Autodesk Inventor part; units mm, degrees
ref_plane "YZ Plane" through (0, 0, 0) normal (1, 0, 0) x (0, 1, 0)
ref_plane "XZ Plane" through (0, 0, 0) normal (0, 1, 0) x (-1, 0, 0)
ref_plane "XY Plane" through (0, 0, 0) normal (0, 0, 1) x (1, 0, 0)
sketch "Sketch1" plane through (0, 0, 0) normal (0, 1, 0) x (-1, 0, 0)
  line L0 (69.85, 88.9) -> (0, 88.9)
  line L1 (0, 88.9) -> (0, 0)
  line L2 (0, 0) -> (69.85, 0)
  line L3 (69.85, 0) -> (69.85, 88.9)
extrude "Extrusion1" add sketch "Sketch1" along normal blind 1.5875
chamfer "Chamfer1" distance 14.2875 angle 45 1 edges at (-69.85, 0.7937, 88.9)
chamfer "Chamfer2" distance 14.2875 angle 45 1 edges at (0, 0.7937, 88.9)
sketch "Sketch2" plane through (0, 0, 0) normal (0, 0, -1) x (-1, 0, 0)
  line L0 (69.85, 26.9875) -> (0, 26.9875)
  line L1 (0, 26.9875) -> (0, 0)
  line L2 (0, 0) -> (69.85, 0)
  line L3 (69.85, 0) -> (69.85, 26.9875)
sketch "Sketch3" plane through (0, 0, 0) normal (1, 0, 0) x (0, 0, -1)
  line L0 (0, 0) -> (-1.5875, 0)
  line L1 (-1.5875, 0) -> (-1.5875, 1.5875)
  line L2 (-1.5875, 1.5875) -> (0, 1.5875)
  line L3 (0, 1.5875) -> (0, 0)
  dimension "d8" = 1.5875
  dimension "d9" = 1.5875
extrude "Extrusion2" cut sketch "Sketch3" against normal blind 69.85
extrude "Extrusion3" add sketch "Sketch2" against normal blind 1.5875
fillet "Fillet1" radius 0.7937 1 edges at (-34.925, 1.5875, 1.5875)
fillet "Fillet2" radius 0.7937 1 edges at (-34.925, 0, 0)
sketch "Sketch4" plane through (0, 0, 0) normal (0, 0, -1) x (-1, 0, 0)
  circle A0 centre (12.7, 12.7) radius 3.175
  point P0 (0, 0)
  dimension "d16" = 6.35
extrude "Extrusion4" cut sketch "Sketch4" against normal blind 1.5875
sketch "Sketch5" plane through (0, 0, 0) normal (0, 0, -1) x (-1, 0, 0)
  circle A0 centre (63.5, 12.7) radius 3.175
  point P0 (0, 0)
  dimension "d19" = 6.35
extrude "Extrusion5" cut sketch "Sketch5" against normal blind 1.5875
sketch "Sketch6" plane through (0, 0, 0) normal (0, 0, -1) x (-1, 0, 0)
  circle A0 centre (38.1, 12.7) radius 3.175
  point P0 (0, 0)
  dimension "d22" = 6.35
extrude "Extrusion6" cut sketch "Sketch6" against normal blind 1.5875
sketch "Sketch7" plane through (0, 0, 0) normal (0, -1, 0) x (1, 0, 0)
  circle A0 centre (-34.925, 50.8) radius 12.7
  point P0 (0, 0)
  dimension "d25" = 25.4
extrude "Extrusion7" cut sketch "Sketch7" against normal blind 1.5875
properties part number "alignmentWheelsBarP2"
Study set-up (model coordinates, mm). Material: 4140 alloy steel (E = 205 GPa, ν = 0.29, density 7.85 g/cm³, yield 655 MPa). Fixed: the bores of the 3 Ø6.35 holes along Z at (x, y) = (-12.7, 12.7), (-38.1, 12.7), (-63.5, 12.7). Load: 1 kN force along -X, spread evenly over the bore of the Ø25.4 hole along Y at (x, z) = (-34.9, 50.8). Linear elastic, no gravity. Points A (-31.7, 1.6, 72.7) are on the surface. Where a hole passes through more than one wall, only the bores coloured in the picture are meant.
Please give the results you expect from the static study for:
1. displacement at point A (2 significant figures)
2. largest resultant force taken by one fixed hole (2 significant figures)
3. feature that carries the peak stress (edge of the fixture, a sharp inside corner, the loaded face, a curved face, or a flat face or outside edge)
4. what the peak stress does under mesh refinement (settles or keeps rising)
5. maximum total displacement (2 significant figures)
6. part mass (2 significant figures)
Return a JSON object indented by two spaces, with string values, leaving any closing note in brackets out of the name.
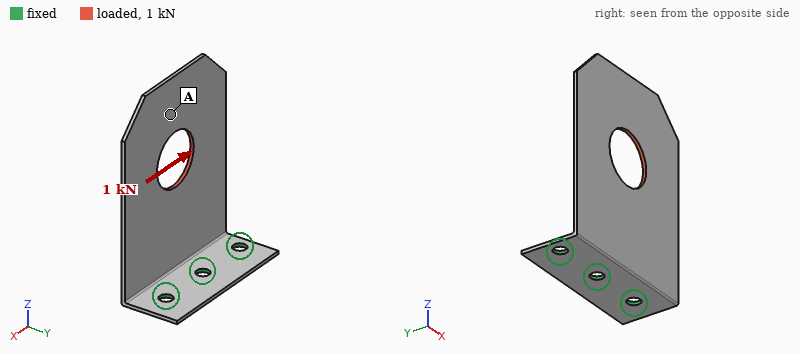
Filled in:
{
  "displacement at point A": "0.47 mm",
  "largest resultant force taken by one fixed hole": "1.0 kN",
  "feature that carries the peak stress": "edge of the fixture",
  "what the peak stress does under mesh refinement": "keeps rising",
  "maximum total displacement": "0.72 mm",
  "part mass": "89 g"
}
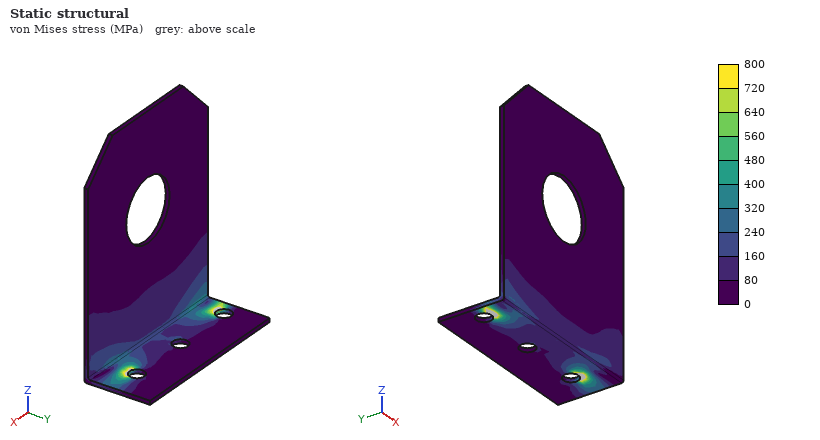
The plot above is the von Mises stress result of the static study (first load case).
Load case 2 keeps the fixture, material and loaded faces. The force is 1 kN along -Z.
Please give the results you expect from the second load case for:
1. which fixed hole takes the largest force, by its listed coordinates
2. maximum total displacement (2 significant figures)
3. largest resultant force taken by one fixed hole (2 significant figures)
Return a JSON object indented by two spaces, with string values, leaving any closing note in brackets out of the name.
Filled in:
{
  "which fixed hole takes the largest force, by its listed coordinates": "(-12.7, 12.7)",
  "maximum total displacement": "0.93 mm",
  "largest resultant force taken by one fixed hole": "390 N"
}
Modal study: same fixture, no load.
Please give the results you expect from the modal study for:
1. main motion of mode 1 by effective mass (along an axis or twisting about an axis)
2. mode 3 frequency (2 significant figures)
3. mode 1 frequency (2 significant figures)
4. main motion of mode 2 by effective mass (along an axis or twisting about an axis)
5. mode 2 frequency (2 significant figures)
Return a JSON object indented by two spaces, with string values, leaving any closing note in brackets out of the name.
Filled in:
{
  "main motion of mode 1 by effective mass": "along Y",
  "mode 3 frequency": "900 Hz",
  "mode 1 frequency": "160 Hz",
  "main motion of mode 2 by effective mass": "twisting about Z",
  "mode 2 frequency": "490 Hz"
}
